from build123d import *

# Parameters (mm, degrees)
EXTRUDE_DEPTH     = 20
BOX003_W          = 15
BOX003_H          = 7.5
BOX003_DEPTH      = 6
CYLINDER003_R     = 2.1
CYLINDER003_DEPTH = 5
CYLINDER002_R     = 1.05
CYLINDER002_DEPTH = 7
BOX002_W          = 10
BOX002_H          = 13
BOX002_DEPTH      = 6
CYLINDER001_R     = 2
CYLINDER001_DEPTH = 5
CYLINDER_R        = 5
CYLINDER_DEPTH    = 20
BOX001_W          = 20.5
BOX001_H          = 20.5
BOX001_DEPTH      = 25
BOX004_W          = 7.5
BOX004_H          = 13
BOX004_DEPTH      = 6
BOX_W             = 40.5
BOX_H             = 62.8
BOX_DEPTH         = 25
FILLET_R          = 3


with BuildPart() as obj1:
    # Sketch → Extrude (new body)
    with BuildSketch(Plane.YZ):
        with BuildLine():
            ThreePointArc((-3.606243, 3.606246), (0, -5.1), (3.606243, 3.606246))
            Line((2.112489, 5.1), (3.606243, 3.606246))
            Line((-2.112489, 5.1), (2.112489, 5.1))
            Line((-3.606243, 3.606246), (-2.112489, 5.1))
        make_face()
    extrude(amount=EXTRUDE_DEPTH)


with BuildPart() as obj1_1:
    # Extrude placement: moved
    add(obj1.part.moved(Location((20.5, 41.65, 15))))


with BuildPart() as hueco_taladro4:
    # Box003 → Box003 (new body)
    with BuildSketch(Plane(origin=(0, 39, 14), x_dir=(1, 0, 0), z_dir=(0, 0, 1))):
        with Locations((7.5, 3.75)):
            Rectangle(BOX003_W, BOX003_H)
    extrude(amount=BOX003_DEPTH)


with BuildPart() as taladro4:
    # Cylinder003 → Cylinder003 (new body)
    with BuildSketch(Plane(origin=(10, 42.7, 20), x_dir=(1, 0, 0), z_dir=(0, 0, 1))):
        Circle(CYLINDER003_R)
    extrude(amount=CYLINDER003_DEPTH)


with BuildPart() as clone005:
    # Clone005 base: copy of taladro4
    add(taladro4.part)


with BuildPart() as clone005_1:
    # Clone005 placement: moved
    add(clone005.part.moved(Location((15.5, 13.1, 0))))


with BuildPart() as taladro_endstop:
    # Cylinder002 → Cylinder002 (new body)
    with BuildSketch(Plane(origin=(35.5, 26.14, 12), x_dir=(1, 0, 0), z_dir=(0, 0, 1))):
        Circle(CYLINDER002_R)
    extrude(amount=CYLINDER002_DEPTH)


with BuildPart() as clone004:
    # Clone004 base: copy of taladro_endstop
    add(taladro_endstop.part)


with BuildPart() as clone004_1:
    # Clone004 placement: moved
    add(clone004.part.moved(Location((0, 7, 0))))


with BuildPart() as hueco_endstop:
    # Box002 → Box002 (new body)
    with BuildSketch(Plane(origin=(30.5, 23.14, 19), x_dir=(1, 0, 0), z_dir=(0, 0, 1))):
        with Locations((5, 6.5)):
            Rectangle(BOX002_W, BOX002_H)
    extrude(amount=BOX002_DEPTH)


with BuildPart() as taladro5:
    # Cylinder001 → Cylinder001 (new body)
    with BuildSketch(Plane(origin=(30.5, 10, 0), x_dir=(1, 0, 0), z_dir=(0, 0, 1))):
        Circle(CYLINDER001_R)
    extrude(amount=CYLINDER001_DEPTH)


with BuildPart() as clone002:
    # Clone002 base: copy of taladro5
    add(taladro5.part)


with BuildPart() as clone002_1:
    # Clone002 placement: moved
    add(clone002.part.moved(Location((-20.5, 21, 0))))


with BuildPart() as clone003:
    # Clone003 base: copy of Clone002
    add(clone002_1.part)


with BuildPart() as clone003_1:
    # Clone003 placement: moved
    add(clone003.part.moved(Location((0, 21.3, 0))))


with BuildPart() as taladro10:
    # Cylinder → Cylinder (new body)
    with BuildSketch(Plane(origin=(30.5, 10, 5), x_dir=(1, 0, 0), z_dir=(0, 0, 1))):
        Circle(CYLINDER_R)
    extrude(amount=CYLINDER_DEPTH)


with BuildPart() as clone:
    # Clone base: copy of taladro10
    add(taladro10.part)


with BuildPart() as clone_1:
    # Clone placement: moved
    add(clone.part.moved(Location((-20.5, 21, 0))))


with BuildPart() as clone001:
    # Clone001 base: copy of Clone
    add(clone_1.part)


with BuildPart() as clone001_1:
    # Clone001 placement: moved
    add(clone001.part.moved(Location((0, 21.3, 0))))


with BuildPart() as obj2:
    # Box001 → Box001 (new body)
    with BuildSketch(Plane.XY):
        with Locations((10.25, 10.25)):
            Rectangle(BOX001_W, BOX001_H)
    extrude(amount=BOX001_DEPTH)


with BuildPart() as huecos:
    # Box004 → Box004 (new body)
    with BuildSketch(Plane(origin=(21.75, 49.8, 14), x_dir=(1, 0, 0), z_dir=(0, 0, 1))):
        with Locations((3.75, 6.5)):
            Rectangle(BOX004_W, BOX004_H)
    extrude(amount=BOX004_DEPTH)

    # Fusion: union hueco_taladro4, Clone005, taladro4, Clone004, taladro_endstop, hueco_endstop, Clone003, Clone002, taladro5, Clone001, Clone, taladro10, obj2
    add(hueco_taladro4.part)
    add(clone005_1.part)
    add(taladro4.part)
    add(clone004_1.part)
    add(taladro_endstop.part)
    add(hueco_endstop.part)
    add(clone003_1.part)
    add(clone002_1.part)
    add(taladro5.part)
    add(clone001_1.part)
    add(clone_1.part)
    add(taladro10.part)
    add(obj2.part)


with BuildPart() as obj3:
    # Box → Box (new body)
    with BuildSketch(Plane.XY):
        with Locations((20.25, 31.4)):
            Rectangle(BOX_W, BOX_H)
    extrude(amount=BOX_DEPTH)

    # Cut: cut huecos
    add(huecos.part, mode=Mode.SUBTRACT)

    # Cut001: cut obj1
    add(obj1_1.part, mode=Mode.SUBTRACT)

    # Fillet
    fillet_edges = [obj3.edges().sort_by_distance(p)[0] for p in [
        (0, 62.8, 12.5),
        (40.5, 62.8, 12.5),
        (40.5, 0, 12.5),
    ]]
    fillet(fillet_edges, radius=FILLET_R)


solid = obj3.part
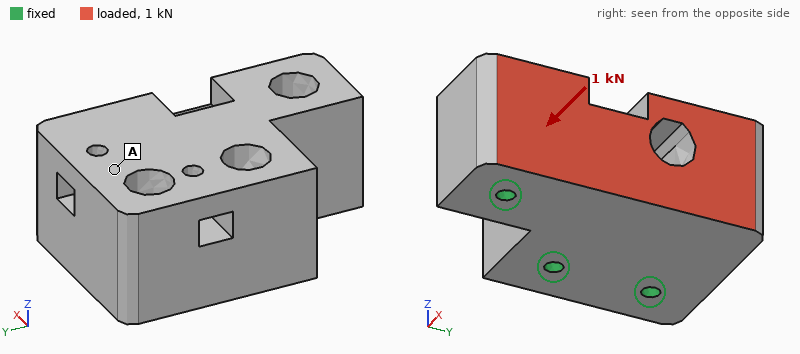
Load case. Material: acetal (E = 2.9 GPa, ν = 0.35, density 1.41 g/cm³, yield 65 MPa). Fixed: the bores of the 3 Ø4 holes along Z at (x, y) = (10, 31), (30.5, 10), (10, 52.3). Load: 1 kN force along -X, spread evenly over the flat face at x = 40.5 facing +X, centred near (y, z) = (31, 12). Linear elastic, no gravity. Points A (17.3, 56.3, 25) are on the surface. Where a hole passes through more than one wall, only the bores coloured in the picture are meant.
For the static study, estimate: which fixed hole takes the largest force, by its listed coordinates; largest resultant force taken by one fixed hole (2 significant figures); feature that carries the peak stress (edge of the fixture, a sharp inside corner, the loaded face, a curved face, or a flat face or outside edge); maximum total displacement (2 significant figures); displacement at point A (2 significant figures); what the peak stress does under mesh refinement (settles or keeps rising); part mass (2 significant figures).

(10, 31)
570 N
edge of the fixture
0.26 mm
0.16 mm
keeps rising
62 g
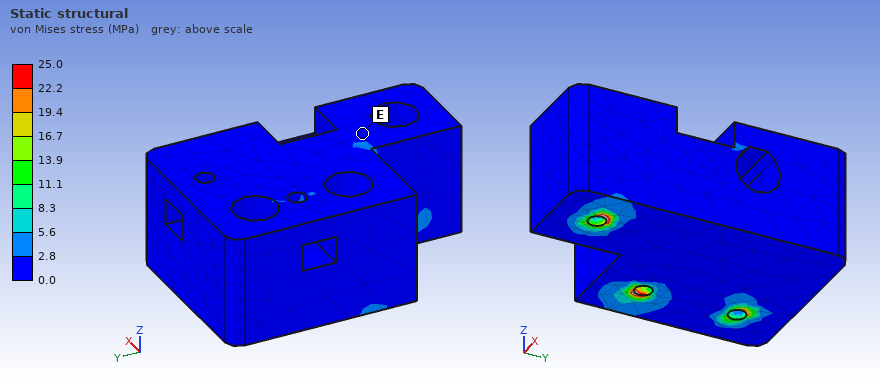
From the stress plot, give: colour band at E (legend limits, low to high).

0.0 to 2.8 MPa
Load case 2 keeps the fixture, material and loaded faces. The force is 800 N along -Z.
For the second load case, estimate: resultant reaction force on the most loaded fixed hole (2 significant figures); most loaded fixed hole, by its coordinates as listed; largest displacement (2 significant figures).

820 N
(30.5, 10)
0.54 mm
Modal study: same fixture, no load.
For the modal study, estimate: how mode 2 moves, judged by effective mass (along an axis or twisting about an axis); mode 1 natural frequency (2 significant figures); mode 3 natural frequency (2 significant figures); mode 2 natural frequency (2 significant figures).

along Y
1300 Hz
3800 Hz
3500 Hz
